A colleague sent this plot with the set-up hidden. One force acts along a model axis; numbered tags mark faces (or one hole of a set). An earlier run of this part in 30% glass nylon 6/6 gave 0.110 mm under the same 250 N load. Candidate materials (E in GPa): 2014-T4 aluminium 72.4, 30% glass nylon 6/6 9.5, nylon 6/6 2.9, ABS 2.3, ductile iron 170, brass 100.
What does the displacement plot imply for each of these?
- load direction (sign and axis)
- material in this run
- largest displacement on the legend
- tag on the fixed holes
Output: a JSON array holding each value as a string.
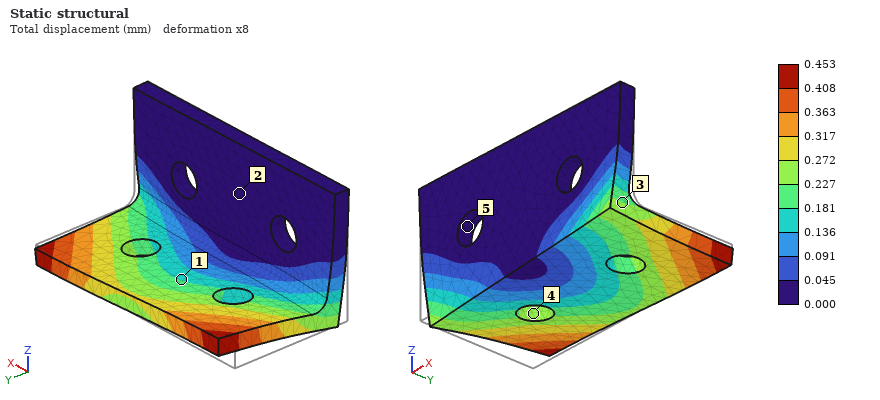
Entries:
["+X", "ABS", "0.453 mm", "5"]
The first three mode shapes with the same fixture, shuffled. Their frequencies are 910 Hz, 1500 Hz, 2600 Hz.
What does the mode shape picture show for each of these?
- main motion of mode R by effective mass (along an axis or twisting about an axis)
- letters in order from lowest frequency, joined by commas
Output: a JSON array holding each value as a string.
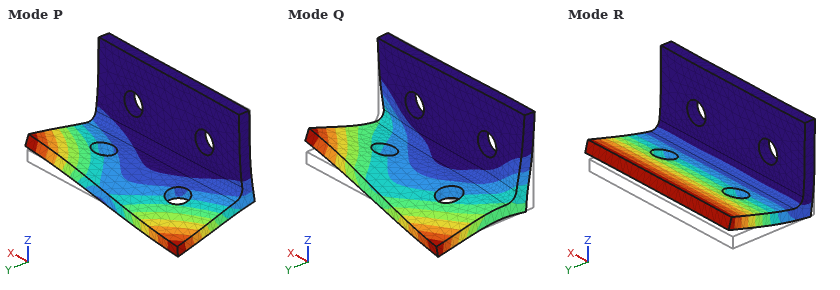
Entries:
["along Z", "R, P, Q"]
